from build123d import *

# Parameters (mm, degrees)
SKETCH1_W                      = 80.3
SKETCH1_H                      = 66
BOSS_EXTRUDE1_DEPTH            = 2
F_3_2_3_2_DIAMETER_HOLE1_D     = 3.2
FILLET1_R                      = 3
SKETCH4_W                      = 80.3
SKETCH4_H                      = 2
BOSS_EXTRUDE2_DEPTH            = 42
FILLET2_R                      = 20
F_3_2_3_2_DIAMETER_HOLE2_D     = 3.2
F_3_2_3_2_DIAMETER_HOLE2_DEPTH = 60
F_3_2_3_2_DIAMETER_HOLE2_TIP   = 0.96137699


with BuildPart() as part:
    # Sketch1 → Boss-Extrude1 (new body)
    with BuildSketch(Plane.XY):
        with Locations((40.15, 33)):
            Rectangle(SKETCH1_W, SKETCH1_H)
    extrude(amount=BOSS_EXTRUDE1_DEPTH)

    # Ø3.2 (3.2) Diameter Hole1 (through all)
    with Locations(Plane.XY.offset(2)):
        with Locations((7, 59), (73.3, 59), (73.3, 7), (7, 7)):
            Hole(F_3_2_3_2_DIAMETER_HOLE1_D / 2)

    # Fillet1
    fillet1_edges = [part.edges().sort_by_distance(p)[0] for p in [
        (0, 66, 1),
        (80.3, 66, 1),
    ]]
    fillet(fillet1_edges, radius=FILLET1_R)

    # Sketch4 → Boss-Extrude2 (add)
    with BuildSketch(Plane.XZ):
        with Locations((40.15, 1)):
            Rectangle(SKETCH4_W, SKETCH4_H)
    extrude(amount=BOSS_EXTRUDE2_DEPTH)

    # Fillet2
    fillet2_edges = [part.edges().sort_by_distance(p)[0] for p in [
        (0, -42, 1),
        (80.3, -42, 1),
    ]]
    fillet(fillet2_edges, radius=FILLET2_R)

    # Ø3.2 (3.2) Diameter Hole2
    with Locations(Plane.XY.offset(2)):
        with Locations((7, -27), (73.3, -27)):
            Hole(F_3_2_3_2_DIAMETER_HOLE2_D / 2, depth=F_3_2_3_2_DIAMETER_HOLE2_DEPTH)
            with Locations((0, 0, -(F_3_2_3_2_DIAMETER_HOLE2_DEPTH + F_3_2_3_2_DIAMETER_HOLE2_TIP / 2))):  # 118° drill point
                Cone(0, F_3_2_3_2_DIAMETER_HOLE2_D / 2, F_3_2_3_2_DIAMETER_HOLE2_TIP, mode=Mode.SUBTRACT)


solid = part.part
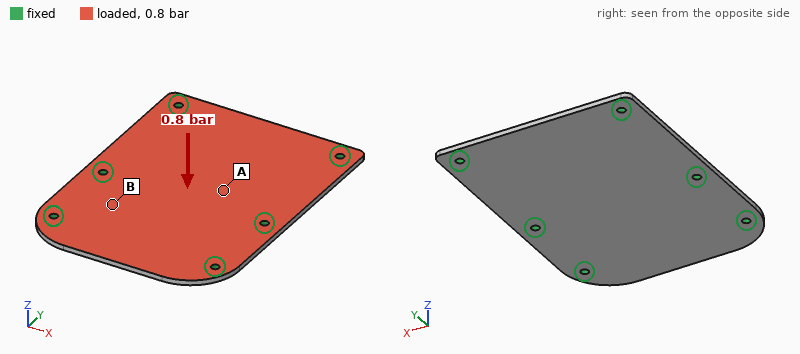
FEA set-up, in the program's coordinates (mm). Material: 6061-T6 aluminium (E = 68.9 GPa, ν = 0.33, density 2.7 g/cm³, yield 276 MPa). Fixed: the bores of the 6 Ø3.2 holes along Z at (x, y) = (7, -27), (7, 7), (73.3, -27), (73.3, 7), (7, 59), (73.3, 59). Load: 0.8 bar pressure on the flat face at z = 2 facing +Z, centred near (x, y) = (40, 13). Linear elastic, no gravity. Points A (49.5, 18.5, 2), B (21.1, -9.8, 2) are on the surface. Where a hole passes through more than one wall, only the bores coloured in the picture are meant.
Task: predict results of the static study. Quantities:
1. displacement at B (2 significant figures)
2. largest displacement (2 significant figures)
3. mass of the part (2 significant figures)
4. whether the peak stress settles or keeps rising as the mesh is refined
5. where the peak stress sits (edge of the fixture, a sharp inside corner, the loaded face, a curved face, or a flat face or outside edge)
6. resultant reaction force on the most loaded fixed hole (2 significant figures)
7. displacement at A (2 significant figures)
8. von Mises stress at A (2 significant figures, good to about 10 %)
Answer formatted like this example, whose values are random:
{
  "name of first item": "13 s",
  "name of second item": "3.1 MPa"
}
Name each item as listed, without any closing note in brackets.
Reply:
{
  "displacement at B": "0.057 mm",
  "largest displacement": "0.15 mm",
  "mass of the part": "46 g",
  "whether the peak stress settles or keeps rising as the mesh is refined": "keeps rising",
  "where the peak stress sits": "edge of the fixture",
  "resultant reaction force on the most loaded fixed hole": "140 N",
  "displacement at A": "0.12 mm",
  "von Mises stress at A": "19 MPa"
}
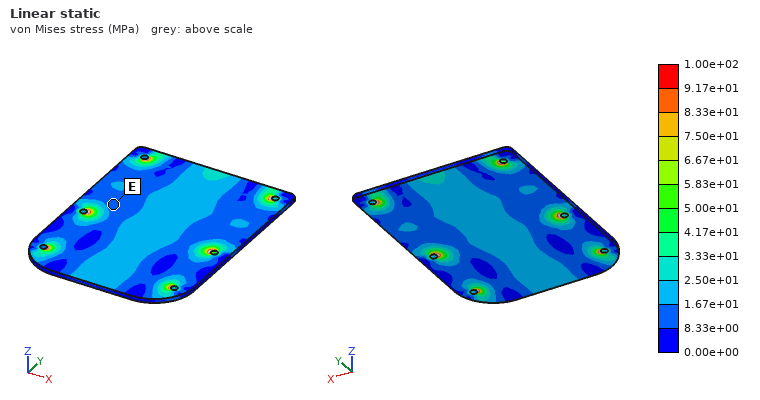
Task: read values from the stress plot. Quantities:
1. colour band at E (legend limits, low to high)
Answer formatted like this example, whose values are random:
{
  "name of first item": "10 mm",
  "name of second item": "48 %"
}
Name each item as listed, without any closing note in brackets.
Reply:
{
  "colour band at E": "8.33e+00 to 1.67e+01 MPa"
}
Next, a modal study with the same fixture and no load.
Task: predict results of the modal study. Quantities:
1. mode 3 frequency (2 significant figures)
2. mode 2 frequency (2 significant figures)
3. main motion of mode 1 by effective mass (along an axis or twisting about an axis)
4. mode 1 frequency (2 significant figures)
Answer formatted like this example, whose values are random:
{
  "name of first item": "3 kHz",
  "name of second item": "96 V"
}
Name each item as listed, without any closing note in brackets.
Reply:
{
  "mode 3 frequency": "3000 Hz",
  "mode 2 frequency": "2200 Hz",
  "main motion of mode 1 by effective mass": "along Z",
  "mode 1 frequency": "1900 Hz"
}
